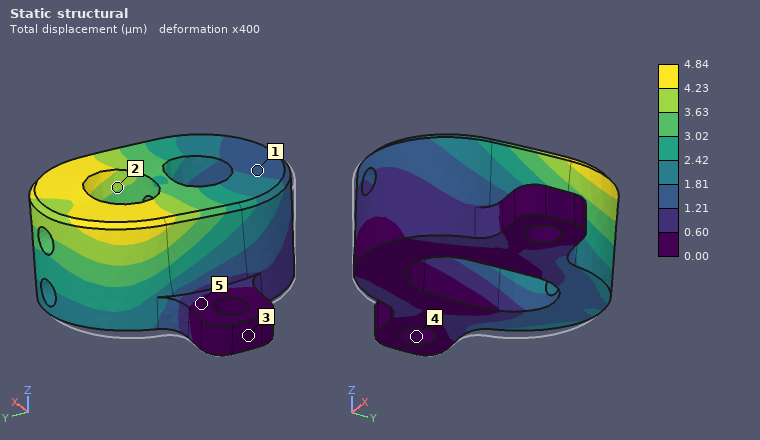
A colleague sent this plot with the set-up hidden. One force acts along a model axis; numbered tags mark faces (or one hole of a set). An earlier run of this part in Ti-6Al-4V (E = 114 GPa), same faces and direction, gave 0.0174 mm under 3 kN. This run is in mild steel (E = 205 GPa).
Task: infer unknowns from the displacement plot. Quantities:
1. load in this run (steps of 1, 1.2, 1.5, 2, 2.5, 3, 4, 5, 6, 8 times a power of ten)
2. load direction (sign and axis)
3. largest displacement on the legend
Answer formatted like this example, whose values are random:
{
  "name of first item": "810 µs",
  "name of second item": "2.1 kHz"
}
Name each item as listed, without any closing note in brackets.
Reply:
{
  "load in this run": "1.5 kN",
  "load direction": "+X",
  "largest displacement on the legend": "4.84 µm"
}
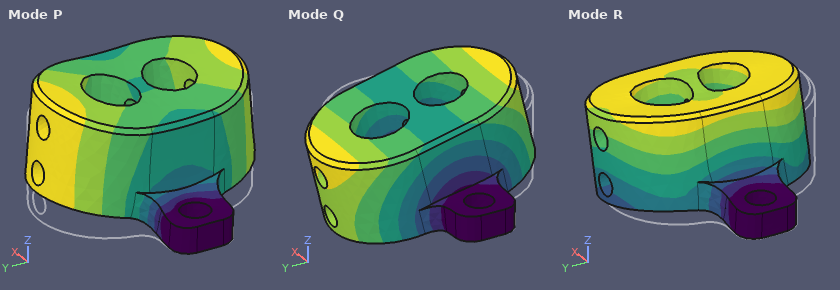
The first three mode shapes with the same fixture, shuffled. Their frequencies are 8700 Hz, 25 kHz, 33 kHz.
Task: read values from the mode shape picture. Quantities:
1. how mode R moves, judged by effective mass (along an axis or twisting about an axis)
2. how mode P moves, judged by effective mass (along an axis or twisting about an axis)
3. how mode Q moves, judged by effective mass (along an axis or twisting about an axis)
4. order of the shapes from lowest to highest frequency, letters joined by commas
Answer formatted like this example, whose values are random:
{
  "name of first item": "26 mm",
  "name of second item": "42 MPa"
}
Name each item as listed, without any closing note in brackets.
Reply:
{
  "how mode R moves, judged by effective mass": "along X",
  "how mode P moves, judged by effective mass": "along Z",
  "how mode Q moves, judged by effective mass": "along Y",
  "order of the shapes from lowest to highest frequency, letters joined by commas": "Q, P, R"
}
